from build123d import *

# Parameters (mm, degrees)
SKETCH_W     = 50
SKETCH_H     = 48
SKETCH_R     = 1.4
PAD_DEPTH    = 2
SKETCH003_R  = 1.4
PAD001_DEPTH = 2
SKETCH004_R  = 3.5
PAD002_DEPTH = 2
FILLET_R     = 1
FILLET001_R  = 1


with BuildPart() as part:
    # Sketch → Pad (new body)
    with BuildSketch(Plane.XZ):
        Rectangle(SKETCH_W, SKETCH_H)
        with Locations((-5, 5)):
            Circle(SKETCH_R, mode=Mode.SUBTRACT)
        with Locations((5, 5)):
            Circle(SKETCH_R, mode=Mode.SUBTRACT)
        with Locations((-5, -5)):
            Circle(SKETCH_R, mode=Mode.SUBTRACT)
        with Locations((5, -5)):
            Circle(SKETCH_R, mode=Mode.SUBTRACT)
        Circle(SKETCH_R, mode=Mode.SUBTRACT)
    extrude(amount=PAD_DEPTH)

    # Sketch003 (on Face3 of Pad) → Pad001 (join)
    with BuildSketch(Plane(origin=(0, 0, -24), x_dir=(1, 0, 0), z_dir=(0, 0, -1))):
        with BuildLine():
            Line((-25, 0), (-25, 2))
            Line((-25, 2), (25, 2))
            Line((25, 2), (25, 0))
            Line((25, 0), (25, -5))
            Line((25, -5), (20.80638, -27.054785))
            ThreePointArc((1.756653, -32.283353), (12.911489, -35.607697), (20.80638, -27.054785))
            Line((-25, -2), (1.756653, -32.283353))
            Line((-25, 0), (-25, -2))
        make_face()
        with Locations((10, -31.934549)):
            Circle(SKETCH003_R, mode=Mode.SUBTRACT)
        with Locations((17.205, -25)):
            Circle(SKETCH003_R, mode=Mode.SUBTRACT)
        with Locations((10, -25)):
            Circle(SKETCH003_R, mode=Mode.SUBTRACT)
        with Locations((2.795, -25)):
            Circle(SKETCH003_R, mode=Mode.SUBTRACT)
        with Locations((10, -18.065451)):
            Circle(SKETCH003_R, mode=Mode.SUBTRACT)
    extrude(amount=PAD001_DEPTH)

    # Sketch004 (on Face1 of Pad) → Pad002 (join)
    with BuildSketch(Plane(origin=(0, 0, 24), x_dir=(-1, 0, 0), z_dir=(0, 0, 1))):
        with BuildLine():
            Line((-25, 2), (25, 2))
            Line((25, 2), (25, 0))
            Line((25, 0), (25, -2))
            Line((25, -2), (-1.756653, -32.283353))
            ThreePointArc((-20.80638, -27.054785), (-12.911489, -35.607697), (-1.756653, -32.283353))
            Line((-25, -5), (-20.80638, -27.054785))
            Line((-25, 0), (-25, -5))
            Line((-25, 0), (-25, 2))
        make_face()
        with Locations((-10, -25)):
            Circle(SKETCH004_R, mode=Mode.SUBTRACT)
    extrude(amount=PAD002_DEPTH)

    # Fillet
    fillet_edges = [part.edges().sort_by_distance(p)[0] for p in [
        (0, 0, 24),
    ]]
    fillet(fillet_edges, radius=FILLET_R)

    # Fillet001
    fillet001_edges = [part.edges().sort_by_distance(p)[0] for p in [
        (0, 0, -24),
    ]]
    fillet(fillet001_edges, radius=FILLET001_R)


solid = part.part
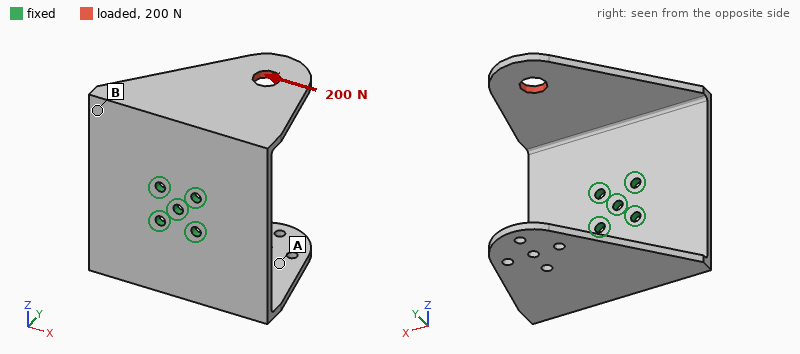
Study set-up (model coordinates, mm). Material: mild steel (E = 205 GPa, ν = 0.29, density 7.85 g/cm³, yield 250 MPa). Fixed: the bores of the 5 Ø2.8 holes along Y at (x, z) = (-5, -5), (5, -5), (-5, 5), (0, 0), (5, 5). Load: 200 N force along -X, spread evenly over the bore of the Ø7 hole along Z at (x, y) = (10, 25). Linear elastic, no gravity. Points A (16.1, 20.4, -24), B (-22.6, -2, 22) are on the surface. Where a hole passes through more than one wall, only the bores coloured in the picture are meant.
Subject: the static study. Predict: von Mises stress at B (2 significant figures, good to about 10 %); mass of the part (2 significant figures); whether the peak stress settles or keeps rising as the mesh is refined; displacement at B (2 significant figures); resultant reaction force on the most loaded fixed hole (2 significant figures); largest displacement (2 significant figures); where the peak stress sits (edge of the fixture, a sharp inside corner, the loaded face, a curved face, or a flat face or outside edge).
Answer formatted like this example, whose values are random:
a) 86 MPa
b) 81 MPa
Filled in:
a) 51 MPa
b) 76 g
c) keeps rising
d) 0.13 mm
e) 380 N
f) 0.25 mm
g) edge of the fixture
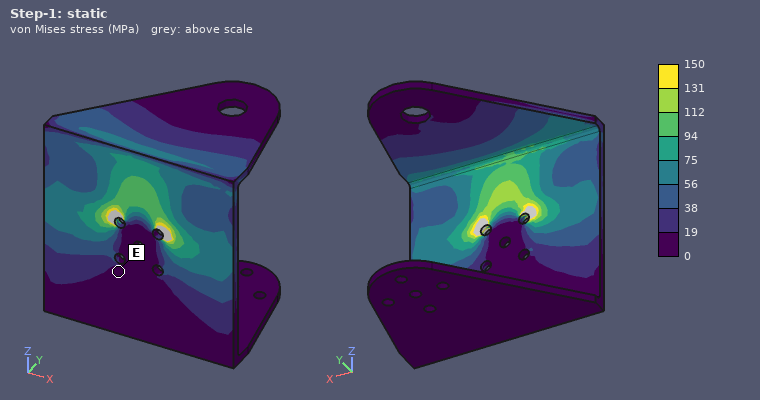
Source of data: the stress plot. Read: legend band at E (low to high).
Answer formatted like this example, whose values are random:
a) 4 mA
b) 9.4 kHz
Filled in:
a) 0 to 19 MPa
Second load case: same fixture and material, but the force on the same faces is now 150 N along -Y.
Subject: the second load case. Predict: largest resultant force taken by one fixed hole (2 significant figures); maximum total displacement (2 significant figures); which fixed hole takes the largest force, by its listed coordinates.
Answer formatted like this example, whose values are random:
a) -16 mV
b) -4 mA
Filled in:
a) 230 N
b) 0.22 mm
c) (5, 5)
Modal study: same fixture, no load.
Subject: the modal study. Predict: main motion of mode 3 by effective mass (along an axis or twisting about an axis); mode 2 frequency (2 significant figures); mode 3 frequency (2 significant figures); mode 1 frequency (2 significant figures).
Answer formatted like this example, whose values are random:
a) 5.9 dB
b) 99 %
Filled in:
a) along X
b) 920 Hz
c) 1500 Hz
d) 910 Hz
